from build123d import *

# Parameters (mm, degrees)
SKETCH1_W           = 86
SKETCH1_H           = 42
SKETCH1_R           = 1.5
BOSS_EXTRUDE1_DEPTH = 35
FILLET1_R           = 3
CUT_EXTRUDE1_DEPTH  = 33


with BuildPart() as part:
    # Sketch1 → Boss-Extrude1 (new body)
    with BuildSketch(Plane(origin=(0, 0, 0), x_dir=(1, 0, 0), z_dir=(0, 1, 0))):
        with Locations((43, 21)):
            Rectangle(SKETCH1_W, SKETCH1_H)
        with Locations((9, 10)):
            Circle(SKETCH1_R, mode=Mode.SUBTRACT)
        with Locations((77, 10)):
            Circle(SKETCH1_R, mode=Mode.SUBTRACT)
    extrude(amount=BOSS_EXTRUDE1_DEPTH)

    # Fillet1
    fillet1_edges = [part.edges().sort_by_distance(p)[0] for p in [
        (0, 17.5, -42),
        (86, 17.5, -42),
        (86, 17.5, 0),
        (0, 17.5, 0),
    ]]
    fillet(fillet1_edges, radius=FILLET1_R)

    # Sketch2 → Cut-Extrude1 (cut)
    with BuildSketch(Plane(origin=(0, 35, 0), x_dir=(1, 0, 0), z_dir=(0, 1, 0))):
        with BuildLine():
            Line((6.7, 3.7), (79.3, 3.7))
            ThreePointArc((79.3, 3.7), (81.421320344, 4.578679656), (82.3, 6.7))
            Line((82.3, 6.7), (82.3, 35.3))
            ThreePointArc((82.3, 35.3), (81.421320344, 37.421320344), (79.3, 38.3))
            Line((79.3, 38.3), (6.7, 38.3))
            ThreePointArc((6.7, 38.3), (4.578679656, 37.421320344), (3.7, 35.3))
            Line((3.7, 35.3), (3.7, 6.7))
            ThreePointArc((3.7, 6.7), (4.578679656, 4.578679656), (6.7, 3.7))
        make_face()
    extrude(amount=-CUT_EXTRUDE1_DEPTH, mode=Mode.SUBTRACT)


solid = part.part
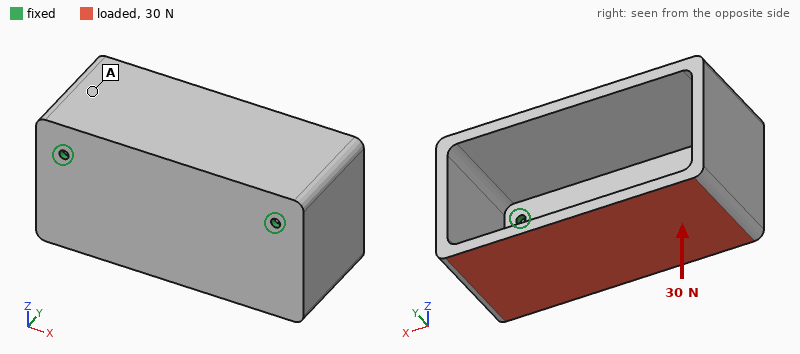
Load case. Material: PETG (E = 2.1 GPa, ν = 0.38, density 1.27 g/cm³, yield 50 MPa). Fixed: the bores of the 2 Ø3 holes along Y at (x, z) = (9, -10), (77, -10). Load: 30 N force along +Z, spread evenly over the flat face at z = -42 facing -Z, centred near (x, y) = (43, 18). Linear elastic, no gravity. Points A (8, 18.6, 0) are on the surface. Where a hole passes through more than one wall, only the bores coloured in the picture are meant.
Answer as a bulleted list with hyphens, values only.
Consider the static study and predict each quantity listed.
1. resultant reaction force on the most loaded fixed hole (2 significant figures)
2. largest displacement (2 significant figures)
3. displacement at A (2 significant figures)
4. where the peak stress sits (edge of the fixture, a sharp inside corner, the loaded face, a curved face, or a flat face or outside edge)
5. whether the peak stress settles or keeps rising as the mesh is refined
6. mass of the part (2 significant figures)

- 15 N
- 0.92 mm
- 0.34 mm
- edge of the fixture
- keeps rising
- 47 g
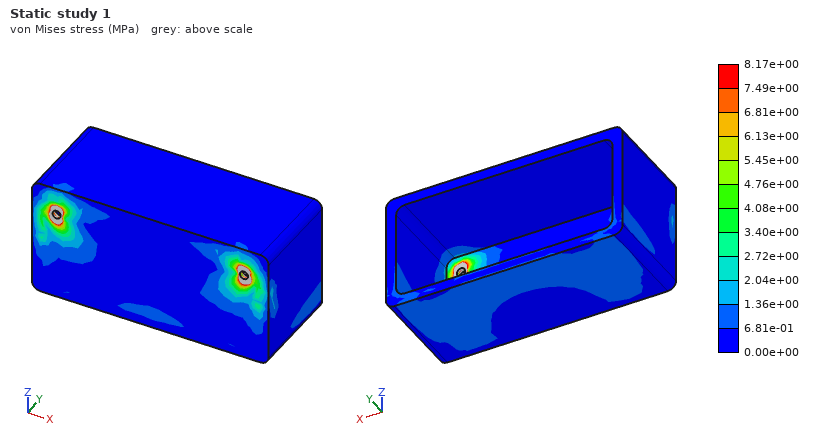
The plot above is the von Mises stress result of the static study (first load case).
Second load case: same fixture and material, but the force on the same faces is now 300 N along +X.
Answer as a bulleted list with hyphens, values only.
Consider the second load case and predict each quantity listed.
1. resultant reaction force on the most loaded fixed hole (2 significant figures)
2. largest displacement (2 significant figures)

- 220 N
- 1.1 mm
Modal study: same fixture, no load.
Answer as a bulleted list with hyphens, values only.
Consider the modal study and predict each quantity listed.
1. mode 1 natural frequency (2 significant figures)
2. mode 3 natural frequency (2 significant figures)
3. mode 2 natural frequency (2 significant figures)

- 150 Hz
- 780 Hz
- 440 Hz
